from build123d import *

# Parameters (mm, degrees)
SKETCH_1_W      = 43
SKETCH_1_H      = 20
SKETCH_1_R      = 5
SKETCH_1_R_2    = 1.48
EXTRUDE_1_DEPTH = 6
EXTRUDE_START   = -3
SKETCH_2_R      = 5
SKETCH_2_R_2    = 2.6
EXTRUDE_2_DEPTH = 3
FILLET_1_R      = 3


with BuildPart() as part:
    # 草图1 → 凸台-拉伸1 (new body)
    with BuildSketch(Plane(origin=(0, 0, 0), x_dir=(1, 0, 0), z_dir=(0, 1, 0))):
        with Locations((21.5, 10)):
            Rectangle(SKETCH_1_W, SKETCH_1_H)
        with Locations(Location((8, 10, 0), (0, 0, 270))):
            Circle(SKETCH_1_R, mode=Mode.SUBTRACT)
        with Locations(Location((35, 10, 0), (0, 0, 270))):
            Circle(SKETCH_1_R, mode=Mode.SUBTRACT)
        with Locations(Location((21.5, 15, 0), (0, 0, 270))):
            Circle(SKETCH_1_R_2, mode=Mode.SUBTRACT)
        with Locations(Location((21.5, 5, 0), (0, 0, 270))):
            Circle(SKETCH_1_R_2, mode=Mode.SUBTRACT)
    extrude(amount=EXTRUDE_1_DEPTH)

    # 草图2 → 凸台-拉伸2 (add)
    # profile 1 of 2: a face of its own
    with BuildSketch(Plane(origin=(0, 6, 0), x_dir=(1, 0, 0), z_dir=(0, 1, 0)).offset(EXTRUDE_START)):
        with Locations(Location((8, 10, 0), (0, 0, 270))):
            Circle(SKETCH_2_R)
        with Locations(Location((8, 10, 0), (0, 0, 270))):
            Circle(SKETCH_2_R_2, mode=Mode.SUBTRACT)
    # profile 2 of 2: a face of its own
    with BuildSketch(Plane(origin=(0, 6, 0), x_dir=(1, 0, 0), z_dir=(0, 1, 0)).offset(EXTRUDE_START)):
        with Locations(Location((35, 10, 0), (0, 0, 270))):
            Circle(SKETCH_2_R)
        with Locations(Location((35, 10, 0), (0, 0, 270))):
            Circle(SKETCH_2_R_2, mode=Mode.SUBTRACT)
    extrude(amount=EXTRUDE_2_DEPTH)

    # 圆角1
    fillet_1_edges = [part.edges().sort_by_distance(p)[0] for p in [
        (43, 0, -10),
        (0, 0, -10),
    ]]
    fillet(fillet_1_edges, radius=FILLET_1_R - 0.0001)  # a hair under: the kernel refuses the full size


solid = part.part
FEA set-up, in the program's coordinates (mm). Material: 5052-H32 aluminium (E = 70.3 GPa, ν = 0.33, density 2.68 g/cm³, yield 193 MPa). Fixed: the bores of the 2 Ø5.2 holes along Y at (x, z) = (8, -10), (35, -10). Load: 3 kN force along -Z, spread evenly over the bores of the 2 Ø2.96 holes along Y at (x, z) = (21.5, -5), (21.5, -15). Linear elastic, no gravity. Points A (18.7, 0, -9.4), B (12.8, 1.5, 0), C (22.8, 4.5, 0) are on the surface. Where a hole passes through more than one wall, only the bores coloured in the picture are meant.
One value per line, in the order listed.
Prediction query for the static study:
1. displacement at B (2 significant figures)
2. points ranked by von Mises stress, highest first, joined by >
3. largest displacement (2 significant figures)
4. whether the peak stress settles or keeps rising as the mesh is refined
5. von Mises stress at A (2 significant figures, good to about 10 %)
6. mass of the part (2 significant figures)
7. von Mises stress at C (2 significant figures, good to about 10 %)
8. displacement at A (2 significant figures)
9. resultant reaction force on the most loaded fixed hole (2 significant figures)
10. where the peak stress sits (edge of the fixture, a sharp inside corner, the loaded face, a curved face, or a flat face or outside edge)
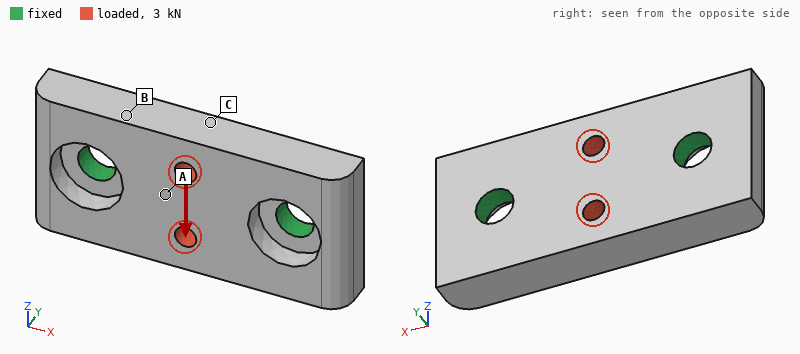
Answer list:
14 µm
C > A > B
20 µm
keeps rising
33 MPa
12 g
58 MPa
15 µm
1.5 kN
edge of the fixture
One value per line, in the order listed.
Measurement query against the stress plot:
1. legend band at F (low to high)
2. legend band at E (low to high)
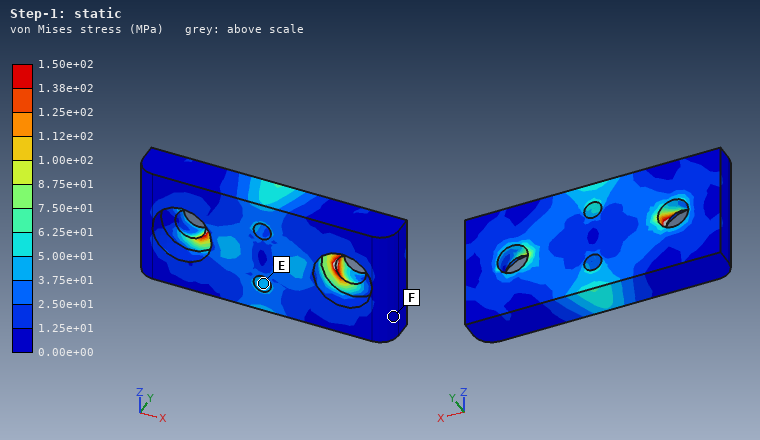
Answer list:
0.00e+00 to 1.25e+01 MPa
3.75e+01 to 5.00e+01 MPa
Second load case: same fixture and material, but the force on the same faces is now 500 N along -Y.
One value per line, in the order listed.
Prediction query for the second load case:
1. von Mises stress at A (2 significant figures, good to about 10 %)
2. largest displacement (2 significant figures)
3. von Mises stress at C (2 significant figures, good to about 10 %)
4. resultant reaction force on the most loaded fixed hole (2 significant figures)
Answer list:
17 MPa
5.6 µm
5.8 MPa
320 N
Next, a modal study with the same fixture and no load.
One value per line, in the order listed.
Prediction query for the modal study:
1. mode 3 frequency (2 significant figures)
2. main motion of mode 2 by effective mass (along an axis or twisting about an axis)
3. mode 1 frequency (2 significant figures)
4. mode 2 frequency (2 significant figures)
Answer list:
27 kHz
along Y
18 kHz
24 kHz
